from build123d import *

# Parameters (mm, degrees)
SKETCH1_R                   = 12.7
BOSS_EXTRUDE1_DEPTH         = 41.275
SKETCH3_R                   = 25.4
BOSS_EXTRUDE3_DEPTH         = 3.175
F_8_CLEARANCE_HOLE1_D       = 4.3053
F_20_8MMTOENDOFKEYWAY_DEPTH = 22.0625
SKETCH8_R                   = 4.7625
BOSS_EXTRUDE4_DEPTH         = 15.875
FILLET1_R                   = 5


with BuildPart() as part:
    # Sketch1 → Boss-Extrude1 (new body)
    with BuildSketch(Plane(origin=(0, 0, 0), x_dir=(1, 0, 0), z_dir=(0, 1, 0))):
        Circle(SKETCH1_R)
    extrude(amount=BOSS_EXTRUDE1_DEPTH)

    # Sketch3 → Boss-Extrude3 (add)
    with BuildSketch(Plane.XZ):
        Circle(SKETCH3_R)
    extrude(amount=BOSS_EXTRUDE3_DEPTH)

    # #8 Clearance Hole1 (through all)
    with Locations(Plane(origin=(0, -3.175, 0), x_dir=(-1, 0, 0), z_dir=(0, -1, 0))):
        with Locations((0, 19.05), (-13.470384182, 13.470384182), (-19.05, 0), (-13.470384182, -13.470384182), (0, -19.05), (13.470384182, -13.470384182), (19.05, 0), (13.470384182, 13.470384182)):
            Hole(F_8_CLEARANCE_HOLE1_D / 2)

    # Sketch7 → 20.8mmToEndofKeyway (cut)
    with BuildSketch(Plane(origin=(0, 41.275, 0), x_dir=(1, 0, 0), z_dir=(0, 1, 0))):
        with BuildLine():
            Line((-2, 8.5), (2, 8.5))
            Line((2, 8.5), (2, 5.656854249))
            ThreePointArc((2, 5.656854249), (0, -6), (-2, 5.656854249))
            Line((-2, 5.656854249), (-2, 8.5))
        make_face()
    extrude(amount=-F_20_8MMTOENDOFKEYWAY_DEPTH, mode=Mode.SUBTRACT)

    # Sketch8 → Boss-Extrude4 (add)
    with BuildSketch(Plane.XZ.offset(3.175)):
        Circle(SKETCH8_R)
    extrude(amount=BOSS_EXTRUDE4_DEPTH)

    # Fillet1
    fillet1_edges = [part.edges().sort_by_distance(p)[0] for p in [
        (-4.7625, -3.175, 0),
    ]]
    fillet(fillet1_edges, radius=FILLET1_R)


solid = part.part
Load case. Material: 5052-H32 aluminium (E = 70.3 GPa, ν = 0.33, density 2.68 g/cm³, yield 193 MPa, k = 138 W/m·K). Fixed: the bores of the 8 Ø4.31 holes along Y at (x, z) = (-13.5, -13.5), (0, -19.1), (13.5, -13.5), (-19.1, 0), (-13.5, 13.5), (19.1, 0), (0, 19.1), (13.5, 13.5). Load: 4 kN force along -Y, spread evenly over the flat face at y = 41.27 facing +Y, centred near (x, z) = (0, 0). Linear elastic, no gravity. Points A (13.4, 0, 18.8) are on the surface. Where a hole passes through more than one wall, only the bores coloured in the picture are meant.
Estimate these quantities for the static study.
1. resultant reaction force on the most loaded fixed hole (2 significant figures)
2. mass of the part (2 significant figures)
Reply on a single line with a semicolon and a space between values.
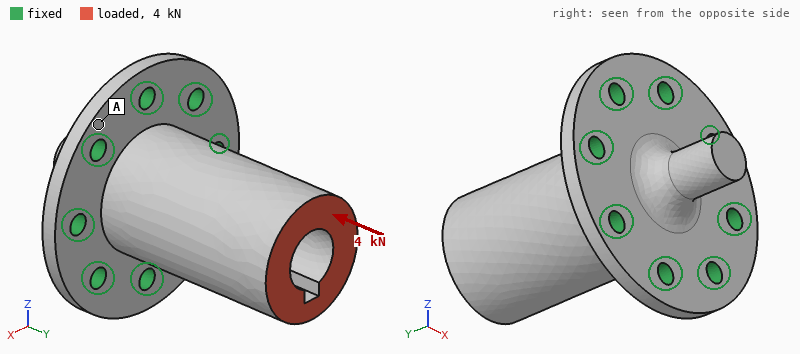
560 N; 69 g
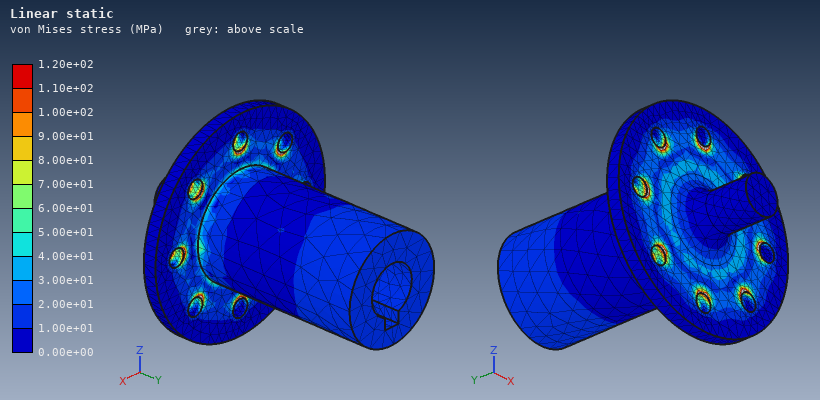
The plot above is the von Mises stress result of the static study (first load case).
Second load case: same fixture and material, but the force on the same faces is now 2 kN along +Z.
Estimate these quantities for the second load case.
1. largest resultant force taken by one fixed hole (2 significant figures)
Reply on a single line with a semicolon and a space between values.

1.5 kN
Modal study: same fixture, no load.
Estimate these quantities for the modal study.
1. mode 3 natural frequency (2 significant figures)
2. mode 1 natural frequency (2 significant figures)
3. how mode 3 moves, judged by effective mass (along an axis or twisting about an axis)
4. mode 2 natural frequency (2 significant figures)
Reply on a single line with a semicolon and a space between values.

12 kHz; 5200 Hz; along Y; 5300 Hz
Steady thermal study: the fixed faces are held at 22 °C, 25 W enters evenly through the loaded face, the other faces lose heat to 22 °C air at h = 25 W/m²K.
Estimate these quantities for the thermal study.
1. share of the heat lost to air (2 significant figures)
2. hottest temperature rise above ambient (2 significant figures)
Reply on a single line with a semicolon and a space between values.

6.6 %; 22 K
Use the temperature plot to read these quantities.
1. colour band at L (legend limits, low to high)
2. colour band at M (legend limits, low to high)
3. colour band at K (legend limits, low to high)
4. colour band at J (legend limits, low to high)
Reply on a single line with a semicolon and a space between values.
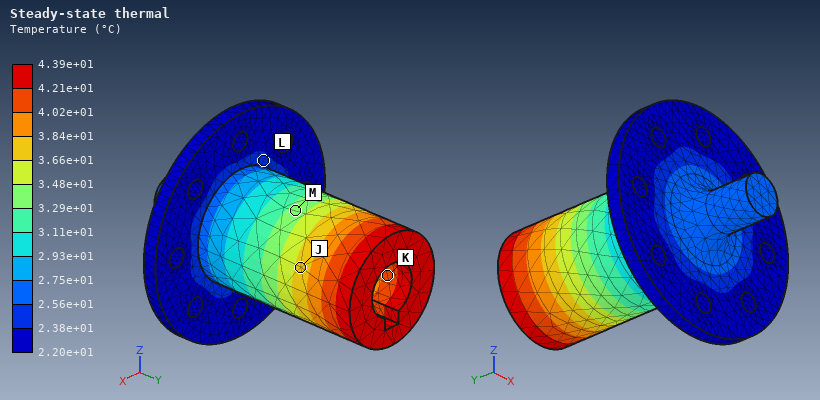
2.38e+01 to 2.56e+01 °C; 3.29e+01 to 3.48e+01 °C; 4.02e+01 to 4.21e+01 °C; 3.66e+01 to 3.84e+01 °C
